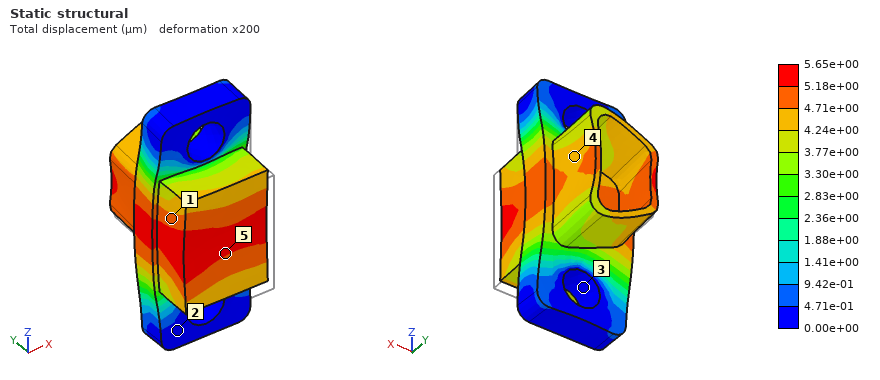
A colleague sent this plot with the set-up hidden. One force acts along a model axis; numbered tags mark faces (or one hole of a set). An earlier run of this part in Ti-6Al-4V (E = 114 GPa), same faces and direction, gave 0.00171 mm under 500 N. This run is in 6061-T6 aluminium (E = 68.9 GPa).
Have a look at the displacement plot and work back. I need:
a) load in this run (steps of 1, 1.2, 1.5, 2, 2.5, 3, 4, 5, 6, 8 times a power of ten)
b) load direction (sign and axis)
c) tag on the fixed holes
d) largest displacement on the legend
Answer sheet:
1 kN
+Y
3
5.65e+00 µm
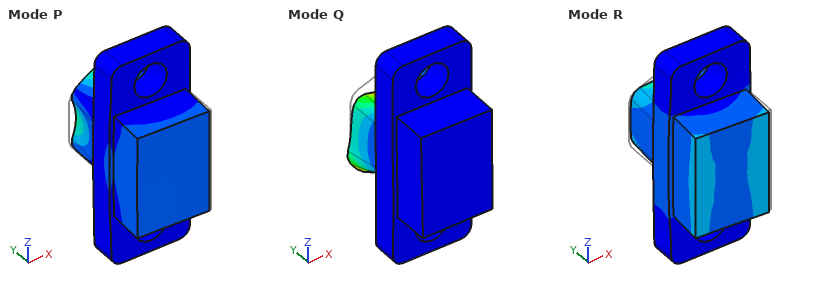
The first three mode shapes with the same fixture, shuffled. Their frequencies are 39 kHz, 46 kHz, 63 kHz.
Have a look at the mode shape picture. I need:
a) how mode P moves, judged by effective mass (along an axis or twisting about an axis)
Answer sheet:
along X
